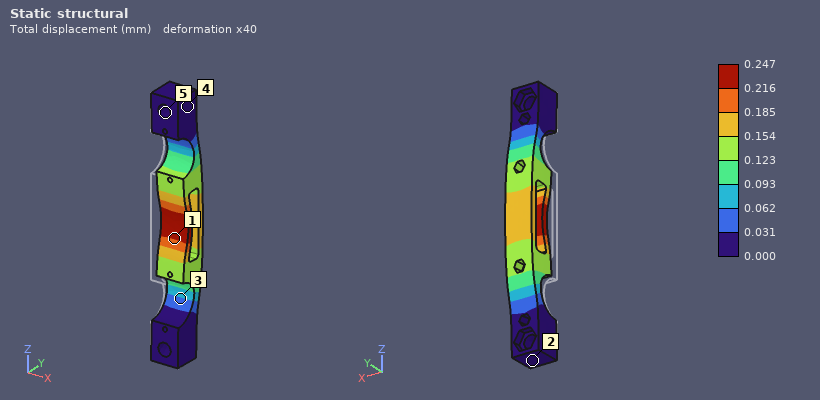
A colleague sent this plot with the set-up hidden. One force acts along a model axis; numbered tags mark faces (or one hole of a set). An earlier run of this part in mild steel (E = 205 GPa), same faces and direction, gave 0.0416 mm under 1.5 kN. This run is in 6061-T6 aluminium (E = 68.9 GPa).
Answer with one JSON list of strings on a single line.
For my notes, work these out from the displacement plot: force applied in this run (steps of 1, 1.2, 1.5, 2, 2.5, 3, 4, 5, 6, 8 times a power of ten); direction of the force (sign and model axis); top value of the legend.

["3 kN", "+Y", "0.247 mm"]
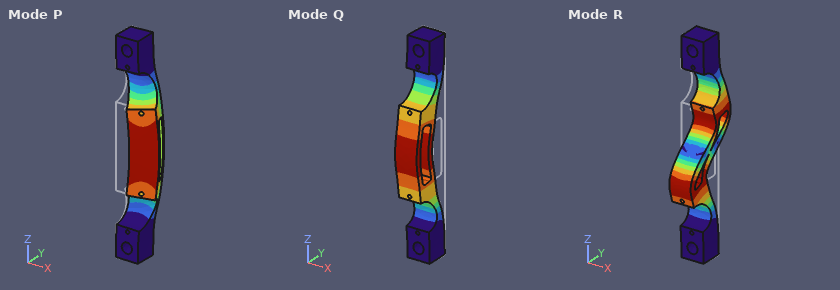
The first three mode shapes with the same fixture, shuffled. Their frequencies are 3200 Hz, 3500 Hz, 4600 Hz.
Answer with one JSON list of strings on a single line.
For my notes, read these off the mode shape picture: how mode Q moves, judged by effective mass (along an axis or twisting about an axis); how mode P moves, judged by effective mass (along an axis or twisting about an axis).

["along Y", "along X"]
